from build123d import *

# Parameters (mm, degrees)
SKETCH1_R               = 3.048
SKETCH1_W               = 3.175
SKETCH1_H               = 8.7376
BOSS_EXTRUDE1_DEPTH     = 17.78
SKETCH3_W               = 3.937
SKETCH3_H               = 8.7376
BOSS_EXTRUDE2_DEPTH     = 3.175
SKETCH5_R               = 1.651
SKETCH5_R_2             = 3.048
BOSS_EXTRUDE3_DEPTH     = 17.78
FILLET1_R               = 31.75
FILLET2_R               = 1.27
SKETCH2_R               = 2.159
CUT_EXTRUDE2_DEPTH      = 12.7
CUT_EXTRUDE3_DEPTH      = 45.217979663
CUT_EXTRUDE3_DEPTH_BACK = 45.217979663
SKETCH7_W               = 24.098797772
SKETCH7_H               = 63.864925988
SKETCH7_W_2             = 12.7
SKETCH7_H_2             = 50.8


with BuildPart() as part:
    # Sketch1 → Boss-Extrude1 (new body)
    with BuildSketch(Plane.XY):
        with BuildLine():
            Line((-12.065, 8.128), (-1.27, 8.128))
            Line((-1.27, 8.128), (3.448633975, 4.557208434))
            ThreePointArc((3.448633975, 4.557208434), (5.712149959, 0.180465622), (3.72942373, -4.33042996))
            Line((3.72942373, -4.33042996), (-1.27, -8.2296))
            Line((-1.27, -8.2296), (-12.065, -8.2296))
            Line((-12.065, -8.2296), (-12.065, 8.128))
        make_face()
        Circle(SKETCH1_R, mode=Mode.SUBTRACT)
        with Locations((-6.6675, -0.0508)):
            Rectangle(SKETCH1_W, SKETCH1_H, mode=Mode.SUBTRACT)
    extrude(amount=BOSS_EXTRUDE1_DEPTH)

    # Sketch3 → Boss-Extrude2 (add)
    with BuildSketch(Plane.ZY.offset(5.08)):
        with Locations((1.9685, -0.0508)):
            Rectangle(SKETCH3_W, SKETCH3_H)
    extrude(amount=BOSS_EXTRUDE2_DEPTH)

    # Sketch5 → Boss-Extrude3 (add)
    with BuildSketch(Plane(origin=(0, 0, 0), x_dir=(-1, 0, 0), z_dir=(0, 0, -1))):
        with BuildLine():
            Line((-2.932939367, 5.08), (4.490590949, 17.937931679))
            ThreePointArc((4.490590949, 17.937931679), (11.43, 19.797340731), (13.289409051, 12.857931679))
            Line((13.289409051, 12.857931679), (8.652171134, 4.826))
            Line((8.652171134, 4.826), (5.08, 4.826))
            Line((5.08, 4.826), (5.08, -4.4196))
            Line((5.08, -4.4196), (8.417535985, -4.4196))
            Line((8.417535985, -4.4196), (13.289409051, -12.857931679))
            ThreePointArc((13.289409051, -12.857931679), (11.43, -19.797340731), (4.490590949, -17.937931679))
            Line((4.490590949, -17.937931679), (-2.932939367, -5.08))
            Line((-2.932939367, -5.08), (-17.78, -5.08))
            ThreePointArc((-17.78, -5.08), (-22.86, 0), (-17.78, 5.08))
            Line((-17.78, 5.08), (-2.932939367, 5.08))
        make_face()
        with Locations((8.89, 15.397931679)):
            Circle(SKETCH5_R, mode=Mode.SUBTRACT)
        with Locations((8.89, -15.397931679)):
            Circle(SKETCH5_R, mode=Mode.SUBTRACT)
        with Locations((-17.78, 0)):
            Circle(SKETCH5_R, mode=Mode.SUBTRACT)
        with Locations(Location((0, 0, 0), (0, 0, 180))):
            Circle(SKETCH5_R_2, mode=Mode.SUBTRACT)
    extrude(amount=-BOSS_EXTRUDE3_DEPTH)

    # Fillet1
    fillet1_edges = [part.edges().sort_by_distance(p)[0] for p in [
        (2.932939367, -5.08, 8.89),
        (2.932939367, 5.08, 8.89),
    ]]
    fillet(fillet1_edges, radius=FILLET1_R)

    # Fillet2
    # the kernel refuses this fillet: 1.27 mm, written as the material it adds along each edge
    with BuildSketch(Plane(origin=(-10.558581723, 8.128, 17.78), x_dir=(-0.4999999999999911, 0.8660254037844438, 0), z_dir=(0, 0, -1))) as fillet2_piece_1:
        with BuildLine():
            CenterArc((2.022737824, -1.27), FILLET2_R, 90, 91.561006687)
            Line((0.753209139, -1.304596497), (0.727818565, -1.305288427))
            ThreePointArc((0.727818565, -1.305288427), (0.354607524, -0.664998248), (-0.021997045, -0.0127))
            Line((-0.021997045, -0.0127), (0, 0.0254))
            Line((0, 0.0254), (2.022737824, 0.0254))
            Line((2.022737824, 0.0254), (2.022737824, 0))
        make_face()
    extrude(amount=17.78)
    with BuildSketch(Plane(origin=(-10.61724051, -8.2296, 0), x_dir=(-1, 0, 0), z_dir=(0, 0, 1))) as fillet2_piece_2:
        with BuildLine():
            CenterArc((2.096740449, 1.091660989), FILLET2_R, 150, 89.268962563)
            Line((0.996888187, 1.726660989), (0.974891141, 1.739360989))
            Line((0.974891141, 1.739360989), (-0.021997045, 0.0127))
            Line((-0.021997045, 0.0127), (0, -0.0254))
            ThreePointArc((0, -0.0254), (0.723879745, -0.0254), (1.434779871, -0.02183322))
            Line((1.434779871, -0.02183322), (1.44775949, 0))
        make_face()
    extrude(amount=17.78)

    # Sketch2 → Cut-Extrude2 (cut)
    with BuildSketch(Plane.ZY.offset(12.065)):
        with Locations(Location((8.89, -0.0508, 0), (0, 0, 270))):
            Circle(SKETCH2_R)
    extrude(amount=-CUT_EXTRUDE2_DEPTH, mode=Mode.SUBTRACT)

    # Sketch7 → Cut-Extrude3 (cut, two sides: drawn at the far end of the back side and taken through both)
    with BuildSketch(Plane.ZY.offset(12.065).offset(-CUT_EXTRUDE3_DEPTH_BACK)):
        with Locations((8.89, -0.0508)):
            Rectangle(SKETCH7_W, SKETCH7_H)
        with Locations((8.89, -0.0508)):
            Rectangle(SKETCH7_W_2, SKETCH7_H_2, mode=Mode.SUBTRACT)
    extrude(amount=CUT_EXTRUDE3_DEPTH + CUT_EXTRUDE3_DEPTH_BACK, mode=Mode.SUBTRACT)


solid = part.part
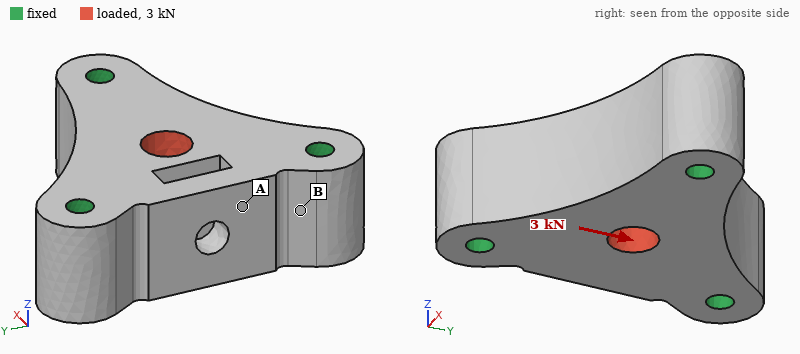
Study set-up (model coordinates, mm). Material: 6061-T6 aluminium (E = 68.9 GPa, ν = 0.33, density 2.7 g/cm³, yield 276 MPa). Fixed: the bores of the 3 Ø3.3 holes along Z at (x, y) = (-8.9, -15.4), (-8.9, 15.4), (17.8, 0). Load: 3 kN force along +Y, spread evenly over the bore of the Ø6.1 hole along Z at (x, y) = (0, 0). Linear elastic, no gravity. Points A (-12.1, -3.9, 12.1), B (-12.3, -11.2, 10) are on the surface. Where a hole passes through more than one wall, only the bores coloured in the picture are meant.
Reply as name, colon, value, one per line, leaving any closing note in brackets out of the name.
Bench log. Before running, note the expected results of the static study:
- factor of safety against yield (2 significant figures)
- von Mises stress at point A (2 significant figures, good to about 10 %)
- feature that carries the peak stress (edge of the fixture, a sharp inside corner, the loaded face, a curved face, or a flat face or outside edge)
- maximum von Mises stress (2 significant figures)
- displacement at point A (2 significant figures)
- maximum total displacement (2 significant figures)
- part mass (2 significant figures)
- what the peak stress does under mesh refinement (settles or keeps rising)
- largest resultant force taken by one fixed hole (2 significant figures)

factor of safety against yield: 5.1
von Mises stress at point A: 13 MPa
feature that carries the peak stress: a curved face
maximum von Mises stress: 54 MPa
displacement at point A: 1.5 µm
maximum total displacement: 5.8 µm
part mass: 24 g
what the peak stress does under mesh refinement: settles
largest resultant force taken by one fixed hole: 1.4 kN
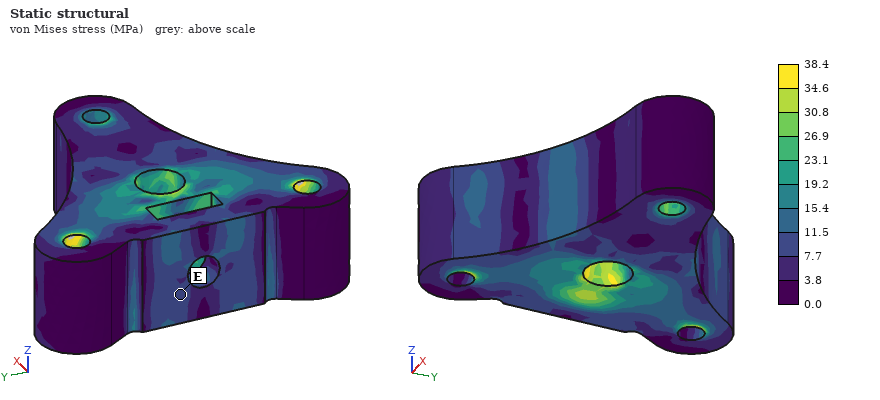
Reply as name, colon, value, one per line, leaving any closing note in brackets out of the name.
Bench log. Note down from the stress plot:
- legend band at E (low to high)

legend band at E: 7.7 to 11.5 MPa
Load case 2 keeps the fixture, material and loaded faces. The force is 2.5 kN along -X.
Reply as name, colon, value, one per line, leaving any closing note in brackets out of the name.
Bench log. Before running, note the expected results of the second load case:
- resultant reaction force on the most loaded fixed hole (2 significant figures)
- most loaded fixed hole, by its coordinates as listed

resultant reaction force on the most loaded fixed hole: 1.4 kN
most loaded fixed hole, by its coordinates as listed: (17.8, 0)
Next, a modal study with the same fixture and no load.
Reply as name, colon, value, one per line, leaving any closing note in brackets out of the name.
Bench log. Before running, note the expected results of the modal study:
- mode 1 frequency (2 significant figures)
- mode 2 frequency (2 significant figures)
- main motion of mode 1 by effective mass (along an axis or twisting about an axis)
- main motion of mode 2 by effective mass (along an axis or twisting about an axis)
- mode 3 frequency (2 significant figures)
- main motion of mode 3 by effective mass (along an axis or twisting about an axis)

mode 1 frequency: 36 kHz
mode 2 frequency: 39 kHz
main motion of mode 1 by effective mass: along Z
main motion of mode 2 by effective mass: along Y
mode 3 frequency: 45 kHz
main motion of mode 3 by effective mass: along X
